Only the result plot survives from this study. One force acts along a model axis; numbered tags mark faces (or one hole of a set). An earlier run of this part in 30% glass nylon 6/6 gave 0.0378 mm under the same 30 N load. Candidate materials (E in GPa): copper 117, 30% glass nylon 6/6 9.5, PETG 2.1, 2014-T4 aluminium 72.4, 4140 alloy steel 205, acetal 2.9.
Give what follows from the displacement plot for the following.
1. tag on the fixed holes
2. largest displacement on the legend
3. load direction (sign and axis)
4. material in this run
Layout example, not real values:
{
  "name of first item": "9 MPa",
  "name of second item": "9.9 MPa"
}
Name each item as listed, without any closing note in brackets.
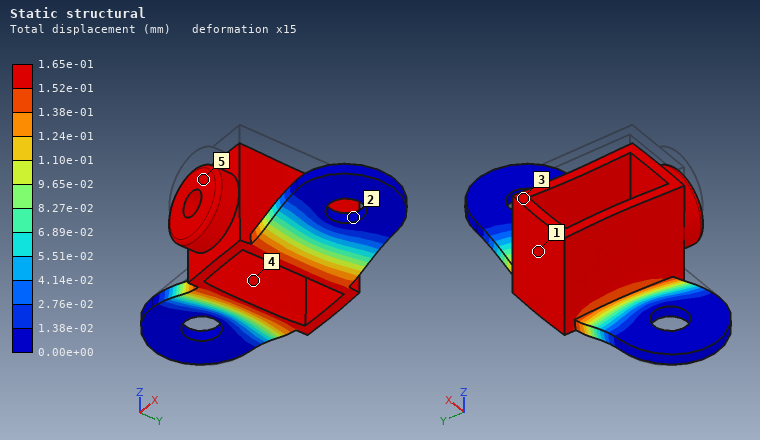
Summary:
{
  "tag on the fixed holes": "2",
  "largest displacement on the legend": "1.65e-01 mm",
  "load direction": "-Z",
  "material in this run": "PETG"
}
